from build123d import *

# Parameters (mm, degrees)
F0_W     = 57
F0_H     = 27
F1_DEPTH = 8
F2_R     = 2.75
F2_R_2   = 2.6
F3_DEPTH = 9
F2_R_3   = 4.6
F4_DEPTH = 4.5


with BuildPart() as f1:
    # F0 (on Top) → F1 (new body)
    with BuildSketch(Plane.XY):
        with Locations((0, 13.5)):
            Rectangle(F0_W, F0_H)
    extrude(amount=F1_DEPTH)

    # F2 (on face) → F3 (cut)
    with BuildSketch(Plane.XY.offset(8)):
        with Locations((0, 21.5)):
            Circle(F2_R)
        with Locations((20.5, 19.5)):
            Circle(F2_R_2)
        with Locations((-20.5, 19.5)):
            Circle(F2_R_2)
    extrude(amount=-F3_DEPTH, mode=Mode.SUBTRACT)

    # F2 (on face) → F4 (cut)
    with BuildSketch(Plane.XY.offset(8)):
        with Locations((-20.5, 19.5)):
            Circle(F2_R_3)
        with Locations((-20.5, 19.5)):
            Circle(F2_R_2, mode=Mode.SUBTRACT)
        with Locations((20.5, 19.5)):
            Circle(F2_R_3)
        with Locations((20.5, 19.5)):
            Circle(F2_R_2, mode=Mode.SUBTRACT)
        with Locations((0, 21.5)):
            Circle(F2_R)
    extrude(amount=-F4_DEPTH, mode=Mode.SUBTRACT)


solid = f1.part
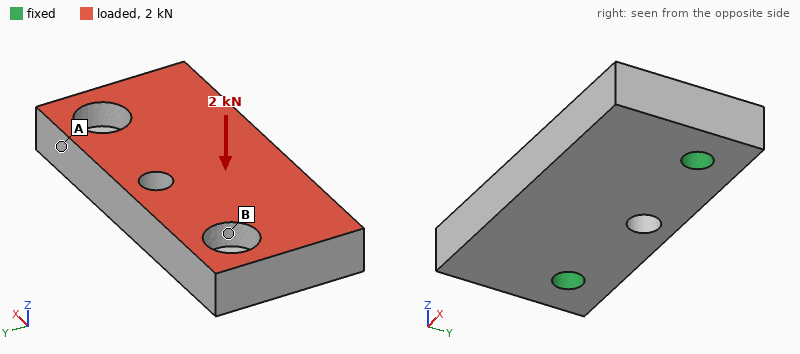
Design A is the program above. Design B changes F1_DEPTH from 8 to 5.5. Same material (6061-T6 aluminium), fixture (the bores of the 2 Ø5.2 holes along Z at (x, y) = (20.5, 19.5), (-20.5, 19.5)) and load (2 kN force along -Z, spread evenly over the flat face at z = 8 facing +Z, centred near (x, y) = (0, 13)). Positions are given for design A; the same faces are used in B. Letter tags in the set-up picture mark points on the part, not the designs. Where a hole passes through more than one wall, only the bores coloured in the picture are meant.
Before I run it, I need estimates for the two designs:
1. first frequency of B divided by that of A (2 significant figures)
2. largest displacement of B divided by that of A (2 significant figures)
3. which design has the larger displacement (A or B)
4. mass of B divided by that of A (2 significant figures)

1.0
1.6
B
0.70
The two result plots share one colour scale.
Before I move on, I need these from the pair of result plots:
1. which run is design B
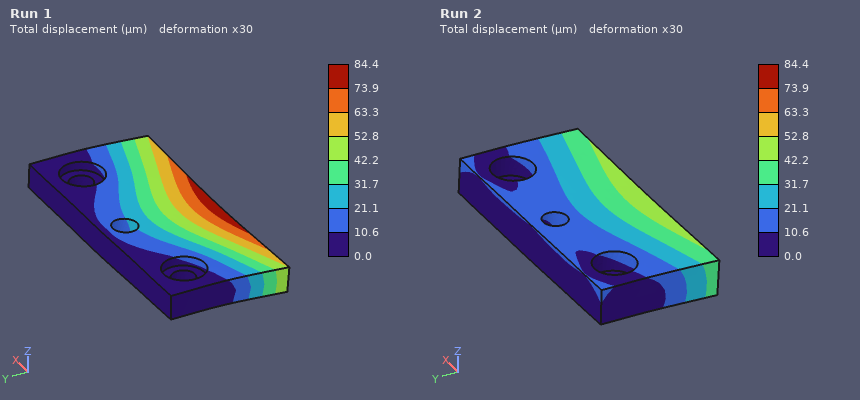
Run 1
